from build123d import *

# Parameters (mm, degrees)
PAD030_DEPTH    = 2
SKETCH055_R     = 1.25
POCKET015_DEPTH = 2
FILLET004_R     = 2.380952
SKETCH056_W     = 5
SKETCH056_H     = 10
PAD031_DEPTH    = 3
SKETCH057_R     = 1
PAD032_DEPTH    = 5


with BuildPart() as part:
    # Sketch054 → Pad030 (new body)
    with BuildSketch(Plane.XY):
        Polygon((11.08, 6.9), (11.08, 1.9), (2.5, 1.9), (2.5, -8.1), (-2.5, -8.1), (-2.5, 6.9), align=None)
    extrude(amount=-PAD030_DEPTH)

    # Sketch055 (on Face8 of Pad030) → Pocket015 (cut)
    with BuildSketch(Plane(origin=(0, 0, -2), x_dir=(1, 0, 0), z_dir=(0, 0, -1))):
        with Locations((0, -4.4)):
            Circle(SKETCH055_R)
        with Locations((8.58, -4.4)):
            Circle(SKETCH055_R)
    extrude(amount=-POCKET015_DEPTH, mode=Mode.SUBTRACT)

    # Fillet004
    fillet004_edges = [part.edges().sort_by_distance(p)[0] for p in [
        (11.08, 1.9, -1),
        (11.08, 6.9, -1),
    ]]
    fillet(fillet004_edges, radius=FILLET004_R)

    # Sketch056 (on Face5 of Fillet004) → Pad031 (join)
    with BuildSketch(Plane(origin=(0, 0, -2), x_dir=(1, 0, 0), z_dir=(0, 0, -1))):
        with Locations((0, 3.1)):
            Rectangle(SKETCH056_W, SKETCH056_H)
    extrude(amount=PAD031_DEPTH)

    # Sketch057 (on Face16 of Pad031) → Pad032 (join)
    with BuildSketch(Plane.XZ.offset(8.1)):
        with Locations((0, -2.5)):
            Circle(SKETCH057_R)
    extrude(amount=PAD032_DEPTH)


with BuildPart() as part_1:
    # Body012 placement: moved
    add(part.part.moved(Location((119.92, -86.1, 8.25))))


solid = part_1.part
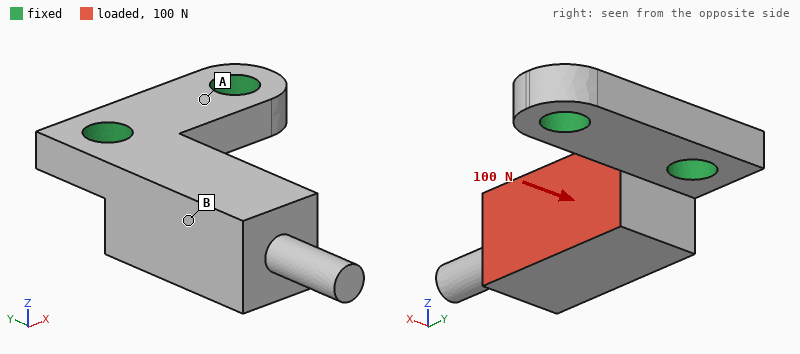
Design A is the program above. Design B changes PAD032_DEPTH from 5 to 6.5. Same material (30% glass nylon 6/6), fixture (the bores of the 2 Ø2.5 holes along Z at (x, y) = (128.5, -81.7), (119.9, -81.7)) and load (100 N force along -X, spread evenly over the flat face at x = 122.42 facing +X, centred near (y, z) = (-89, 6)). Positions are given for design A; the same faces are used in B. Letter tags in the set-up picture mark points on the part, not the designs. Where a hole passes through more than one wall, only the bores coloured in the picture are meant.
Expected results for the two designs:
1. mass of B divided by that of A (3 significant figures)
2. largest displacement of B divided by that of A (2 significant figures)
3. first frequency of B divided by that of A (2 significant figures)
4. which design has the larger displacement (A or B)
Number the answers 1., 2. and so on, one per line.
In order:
1. 1.01
2. 1.1
3. 0.95
4. B
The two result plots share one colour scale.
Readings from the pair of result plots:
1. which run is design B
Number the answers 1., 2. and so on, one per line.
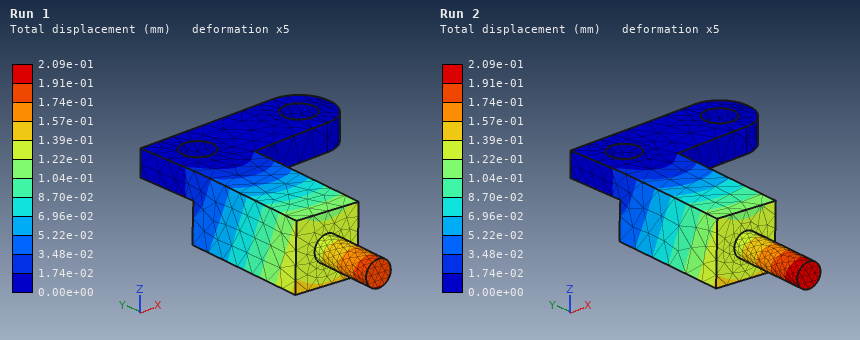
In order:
1. Run 2
